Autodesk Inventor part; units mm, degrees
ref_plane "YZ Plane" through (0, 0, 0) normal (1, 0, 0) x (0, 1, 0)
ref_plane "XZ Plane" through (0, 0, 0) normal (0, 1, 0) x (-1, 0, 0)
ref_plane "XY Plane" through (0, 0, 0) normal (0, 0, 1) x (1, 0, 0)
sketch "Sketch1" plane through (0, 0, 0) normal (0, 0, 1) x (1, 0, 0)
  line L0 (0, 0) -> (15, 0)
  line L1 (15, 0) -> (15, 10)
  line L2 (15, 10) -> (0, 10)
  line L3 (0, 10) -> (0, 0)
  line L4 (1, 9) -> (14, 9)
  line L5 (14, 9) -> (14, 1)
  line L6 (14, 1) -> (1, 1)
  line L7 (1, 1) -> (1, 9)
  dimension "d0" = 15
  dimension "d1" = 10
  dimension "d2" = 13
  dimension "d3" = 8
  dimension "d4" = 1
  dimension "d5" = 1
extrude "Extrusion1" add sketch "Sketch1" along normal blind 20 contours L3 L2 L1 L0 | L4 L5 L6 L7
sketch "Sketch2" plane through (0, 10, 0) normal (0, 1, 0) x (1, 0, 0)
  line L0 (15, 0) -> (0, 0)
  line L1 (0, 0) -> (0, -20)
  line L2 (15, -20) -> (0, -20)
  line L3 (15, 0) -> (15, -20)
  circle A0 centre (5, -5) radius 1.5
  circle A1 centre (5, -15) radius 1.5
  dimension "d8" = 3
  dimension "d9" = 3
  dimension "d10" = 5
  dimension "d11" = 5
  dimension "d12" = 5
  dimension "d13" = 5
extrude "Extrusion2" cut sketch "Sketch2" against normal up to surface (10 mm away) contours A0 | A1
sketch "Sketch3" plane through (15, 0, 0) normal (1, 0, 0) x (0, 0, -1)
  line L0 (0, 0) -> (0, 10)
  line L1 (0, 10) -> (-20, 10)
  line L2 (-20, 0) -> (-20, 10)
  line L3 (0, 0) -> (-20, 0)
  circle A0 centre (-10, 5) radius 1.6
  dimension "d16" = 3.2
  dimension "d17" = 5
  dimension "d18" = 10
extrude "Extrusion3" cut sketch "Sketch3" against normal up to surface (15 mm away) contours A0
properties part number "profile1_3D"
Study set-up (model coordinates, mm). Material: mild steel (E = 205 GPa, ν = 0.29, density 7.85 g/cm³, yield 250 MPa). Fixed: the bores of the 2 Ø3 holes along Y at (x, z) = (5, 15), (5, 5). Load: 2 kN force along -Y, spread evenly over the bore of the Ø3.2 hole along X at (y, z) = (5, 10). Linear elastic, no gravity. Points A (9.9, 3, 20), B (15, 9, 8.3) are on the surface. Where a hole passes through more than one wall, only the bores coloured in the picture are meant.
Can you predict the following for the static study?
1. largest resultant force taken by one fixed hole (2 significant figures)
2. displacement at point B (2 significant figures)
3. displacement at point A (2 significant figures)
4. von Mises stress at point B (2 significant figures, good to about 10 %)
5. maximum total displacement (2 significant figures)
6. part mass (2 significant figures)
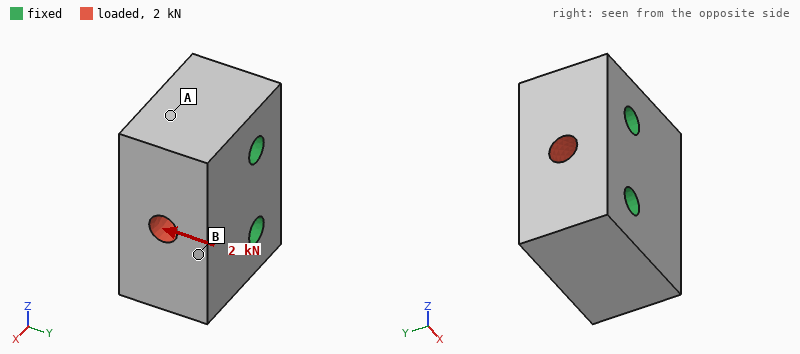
1.0 kN
1.4 µm
0.31 µm
12 MPa
1.5 µm
21 g
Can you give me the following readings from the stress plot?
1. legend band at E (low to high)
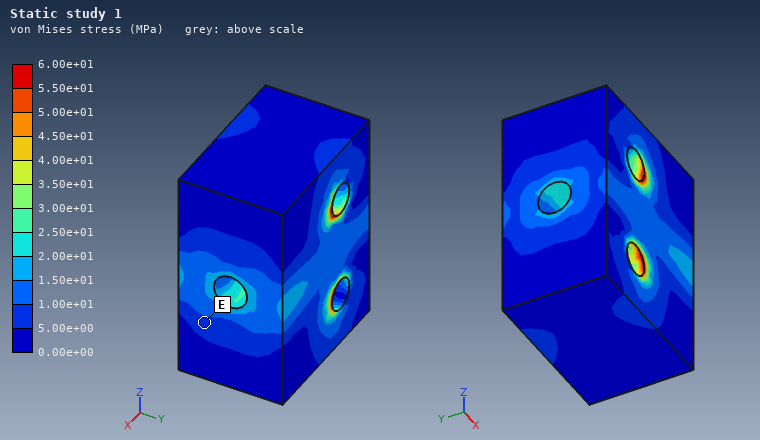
5.00e+00 to 1.00e+01 MPa
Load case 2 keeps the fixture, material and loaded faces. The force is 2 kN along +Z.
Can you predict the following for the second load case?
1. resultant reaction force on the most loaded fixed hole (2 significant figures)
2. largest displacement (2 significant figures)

1.1 kN
0.87 µm
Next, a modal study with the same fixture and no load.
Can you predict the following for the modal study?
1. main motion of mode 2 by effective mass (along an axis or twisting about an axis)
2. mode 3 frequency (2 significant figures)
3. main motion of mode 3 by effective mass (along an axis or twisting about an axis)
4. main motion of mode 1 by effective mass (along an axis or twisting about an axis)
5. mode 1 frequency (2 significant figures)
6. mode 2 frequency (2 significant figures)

along Z
67 kHz
twisting about X
along Y
53 kHz
58 kHz
